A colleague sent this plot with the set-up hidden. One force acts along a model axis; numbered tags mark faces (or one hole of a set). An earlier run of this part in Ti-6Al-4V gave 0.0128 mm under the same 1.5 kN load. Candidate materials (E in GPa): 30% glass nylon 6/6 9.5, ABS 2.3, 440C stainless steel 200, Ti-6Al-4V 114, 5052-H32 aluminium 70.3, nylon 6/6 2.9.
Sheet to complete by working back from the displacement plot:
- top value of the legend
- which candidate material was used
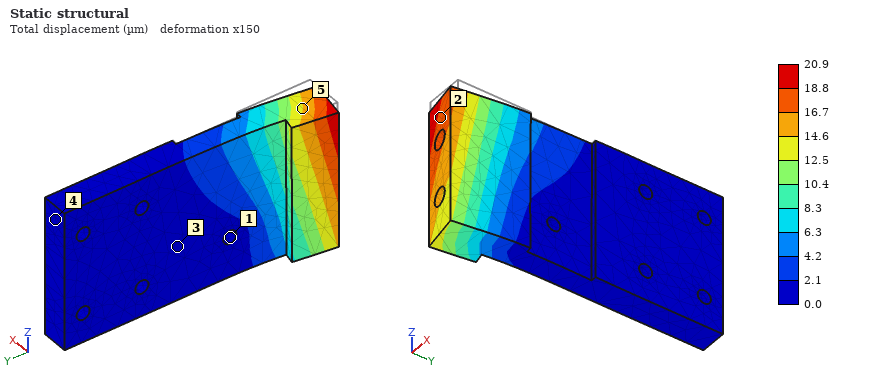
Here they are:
20.9 µm
5052-H32 aluminium
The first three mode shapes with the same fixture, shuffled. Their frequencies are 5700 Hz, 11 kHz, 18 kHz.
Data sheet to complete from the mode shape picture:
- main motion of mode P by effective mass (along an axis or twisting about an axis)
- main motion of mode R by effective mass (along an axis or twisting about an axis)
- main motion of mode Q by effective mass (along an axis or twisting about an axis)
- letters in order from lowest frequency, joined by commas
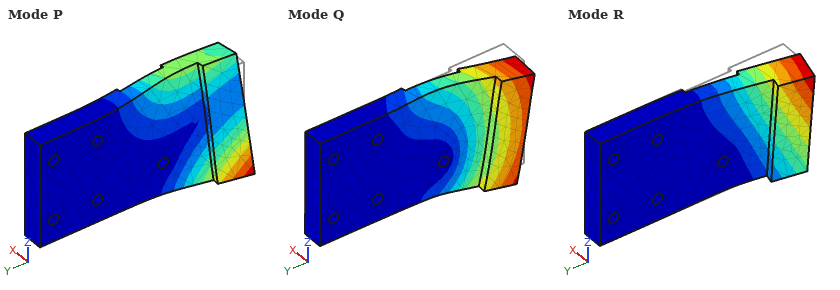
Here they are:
twisting about Y
along X
along Z
R, P, Q
